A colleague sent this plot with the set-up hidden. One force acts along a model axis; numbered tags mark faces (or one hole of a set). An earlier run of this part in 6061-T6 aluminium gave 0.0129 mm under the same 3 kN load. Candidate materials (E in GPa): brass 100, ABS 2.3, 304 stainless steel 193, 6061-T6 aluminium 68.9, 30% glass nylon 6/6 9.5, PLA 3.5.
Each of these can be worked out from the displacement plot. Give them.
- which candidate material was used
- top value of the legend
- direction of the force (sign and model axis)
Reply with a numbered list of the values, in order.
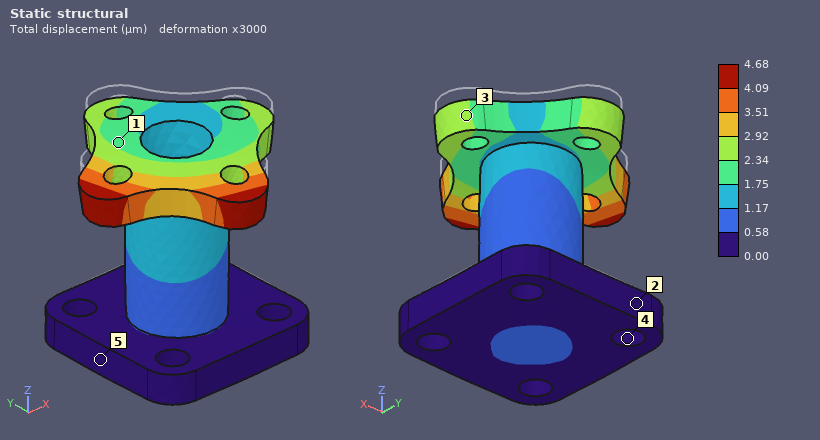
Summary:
1. 304 stainless steel
2. 4.68 µm
3. -Z
